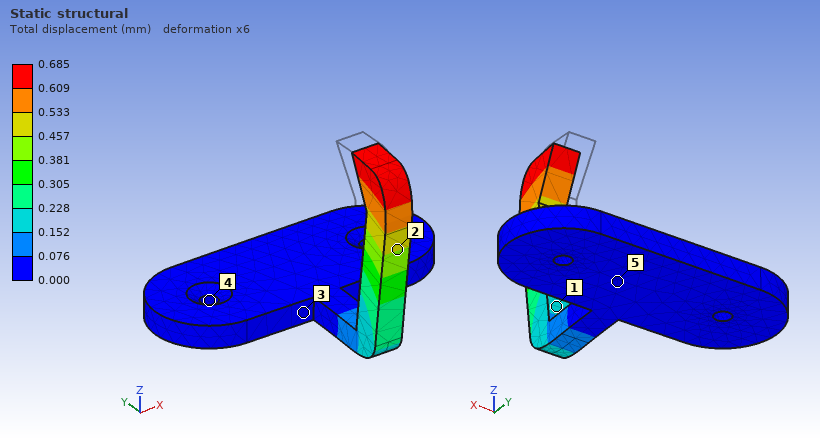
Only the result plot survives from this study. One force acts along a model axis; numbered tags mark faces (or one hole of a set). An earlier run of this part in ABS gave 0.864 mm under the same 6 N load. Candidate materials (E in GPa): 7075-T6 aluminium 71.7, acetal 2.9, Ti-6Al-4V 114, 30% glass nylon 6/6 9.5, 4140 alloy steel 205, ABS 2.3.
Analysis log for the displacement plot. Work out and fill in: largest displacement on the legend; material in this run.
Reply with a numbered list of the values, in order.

1. 0.685 mm
2. acetal
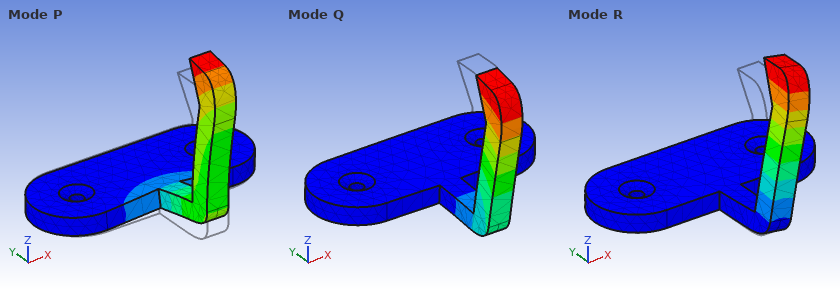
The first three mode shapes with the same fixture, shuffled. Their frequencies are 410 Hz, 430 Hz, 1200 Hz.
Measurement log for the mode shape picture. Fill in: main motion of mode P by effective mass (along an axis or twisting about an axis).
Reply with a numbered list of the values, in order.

1. along Z
